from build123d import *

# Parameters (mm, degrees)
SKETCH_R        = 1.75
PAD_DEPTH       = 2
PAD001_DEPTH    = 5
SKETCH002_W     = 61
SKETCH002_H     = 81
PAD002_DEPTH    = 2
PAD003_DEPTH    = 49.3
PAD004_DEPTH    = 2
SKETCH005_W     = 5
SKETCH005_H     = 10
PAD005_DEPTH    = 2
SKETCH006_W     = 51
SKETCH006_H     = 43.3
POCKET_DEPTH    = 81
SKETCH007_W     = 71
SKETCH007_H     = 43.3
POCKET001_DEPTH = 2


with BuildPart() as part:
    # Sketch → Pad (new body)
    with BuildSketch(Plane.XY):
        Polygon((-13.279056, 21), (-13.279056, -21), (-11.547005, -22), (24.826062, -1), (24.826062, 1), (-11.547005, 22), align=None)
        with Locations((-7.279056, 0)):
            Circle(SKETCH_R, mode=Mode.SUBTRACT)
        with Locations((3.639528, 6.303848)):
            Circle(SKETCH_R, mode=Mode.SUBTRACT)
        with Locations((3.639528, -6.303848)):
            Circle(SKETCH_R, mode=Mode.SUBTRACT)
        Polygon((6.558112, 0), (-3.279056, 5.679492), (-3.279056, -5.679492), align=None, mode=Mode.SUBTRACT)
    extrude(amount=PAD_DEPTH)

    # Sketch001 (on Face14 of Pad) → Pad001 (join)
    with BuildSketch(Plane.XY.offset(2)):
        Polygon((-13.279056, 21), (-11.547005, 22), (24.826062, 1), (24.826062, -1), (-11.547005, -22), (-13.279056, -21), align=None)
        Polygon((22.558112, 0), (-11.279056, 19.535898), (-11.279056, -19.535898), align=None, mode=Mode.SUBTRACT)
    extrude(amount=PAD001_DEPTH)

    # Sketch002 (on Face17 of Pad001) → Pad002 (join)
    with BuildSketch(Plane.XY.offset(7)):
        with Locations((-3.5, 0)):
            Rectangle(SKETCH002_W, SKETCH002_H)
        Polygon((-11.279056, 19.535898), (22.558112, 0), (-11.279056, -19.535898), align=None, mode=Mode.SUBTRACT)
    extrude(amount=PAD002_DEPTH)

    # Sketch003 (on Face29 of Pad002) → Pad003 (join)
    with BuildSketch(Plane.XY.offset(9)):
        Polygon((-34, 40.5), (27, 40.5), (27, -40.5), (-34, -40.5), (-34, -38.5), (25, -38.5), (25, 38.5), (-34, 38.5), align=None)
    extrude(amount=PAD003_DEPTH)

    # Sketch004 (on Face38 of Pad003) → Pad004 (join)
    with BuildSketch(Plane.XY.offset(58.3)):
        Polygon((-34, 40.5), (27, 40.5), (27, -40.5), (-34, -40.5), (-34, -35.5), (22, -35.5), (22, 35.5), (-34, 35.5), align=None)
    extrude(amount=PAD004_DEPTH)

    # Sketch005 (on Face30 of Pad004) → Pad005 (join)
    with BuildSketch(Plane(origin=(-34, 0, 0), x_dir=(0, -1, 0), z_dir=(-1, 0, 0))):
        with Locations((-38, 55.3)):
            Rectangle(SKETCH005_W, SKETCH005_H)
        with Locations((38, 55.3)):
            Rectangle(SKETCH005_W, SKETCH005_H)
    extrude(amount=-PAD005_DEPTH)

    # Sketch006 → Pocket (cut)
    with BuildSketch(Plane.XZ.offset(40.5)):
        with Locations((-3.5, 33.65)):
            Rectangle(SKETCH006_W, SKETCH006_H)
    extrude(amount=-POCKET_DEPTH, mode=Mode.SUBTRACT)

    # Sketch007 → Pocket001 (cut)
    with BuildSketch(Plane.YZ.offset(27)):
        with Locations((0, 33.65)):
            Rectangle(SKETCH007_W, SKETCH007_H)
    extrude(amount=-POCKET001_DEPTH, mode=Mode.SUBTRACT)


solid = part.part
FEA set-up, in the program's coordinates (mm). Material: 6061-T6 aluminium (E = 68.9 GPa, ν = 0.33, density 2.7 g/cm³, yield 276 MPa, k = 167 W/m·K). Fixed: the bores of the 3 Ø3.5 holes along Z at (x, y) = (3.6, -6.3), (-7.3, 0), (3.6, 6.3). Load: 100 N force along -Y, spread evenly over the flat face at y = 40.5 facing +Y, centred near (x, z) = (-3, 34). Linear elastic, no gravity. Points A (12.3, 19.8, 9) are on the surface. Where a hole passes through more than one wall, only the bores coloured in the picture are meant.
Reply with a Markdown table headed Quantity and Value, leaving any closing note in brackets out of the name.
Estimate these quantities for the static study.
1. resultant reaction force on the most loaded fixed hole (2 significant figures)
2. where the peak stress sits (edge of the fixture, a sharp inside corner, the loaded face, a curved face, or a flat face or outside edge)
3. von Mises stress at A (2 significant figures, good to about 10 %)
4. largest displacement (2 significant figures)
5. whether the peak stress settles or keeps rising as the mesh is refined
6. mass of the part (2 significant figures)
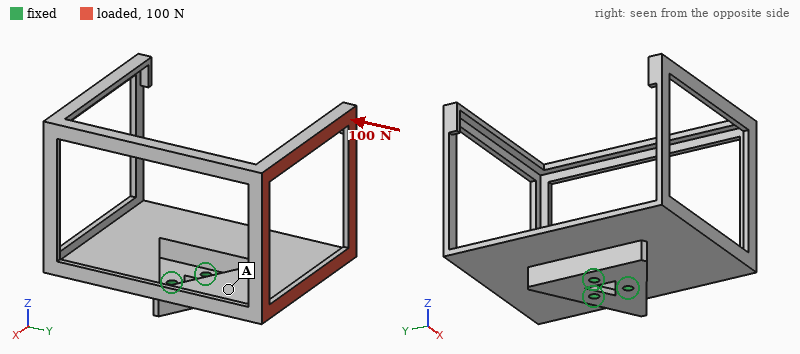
| Quantity | Value |
|---|---|
| resultant reaction force on the most loaded fixed hole | 180 N |
| where the peak stress sits | a sharp inside corner |
| von Mises stress at A | 14 MPa |
| largest displacement | 1.4 mm |
| whether the peak stress settles or keeps rising as the mesh is refined | keeps rising |
| mass of the part | 49 g |
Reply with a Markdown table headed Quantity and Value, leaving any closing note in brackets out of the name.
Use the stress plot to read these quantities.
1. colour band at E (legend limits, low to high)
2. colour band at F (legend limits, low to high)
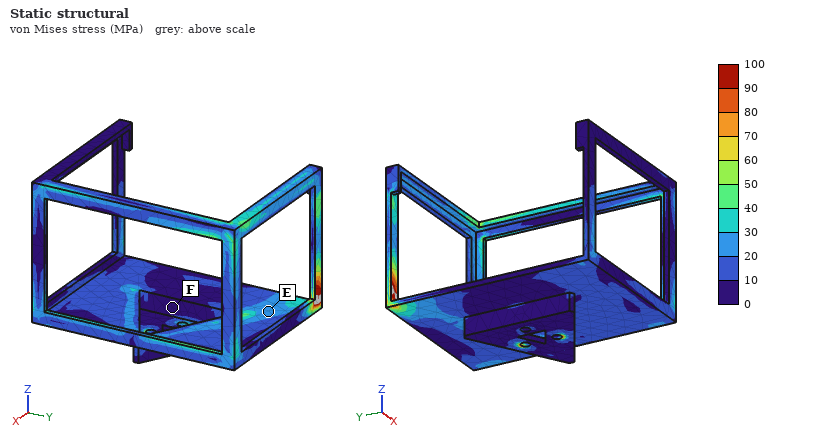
| Quantity | Value |
|---|---|
| colour band at E | 20 to 30 MPa |
| colour band at F | 0 to 10 MPa |
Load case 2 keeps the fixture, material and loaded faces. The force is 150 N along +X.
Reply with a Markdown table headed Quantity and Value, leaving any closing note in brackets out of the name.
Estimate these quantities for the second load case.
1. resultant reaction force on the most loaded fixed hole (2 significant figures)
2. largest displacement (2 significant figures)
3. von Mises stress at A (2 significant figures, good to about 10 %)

| Quantity | Value |
|---|---|
| resultant reaction force on the most loaded fixed hole | 400 N |
| largest displacement | 1.0 mm |
| von Mises stress at A | 26 MPa |
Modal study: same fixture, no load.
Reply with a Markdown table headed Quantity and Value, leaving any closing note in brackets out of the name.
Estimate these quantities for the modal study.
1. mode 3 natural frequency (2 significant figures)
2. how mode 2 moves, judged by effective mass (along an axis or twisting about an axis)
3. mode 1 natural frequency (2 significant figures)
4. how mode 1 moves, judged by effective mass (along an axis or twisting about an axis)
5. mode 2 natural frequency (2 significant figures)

| Quantity | Value |
|---|---|
| mode 3 natural frequency | 730 Hz |
| how mode 2 moves, judged by effective mass | along X |
| mode 1 natural frequency | 410 Hz |
| how mode 1 moves, judged by effective mass | along Y |
| mode 2 natural frequency | 540 Hz |
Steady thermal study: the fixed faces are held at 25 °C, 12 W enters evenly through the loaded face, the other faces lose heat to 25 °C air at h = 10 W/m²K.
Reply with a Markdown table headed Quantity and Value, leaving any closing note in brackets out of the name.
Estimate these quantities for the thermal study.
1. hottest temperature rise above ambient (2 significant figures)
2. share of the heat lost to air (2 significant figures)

| Quantity | Value |
|---|---|
| hottest temperature rise above ambient | 71 K |
| share of the heat lost to air | 23 % |
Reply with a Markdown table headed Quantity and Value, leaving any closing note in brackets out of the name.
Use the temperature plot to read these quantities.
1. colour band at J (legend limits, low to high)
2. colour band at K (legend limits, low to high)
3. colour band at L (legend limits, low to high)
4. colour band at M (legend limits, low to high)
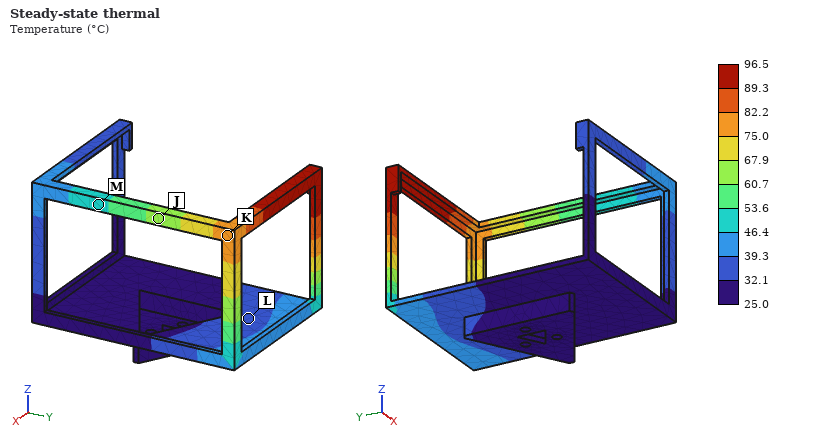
| Quantity | Value |
|---|---|
| colour band at J | 60.7 to 67.9 °C |
| colour band at K | 75.0 to 82.2 °C |
| colour band at L | 32.1 to 39.3 °C |
| colour band at M | 46.4 to 53.6 °C |
